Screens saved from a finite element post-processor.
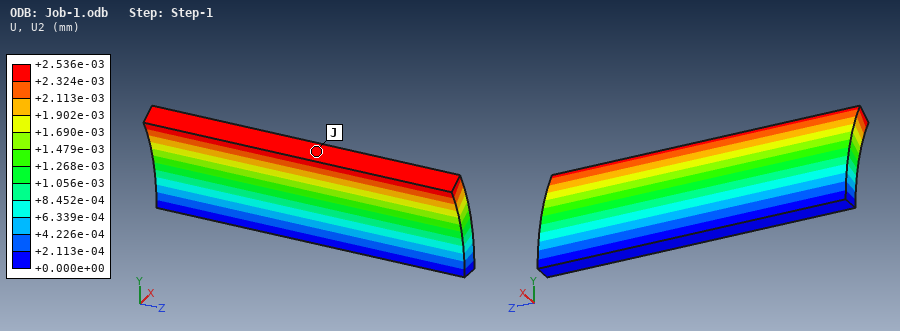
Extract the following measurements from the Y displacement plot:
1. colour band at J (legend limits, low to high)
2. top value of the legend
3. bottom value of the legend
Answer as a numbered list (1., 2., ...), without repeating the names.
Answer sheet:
1. +2.324e-03 to +2.536e-03 mm
2. +2.536e-03 mm
3. +0.000e+00 mm
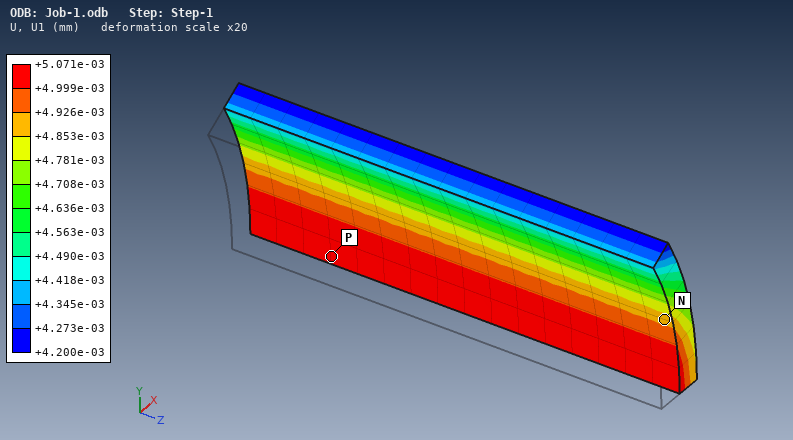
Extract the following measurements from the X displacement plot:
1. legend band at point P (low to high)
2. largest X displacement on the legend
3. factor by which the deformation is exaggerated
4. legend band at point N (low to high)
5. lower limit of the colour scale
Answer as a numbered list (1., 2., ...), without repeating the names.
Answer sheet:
1. +4.999e-03 to +5.071e-03 mm
2. +5.071e-03 mm
3. 20
4. +4.853e-03 to +4.926e-03 mm
5. +4.200e-03 mm
